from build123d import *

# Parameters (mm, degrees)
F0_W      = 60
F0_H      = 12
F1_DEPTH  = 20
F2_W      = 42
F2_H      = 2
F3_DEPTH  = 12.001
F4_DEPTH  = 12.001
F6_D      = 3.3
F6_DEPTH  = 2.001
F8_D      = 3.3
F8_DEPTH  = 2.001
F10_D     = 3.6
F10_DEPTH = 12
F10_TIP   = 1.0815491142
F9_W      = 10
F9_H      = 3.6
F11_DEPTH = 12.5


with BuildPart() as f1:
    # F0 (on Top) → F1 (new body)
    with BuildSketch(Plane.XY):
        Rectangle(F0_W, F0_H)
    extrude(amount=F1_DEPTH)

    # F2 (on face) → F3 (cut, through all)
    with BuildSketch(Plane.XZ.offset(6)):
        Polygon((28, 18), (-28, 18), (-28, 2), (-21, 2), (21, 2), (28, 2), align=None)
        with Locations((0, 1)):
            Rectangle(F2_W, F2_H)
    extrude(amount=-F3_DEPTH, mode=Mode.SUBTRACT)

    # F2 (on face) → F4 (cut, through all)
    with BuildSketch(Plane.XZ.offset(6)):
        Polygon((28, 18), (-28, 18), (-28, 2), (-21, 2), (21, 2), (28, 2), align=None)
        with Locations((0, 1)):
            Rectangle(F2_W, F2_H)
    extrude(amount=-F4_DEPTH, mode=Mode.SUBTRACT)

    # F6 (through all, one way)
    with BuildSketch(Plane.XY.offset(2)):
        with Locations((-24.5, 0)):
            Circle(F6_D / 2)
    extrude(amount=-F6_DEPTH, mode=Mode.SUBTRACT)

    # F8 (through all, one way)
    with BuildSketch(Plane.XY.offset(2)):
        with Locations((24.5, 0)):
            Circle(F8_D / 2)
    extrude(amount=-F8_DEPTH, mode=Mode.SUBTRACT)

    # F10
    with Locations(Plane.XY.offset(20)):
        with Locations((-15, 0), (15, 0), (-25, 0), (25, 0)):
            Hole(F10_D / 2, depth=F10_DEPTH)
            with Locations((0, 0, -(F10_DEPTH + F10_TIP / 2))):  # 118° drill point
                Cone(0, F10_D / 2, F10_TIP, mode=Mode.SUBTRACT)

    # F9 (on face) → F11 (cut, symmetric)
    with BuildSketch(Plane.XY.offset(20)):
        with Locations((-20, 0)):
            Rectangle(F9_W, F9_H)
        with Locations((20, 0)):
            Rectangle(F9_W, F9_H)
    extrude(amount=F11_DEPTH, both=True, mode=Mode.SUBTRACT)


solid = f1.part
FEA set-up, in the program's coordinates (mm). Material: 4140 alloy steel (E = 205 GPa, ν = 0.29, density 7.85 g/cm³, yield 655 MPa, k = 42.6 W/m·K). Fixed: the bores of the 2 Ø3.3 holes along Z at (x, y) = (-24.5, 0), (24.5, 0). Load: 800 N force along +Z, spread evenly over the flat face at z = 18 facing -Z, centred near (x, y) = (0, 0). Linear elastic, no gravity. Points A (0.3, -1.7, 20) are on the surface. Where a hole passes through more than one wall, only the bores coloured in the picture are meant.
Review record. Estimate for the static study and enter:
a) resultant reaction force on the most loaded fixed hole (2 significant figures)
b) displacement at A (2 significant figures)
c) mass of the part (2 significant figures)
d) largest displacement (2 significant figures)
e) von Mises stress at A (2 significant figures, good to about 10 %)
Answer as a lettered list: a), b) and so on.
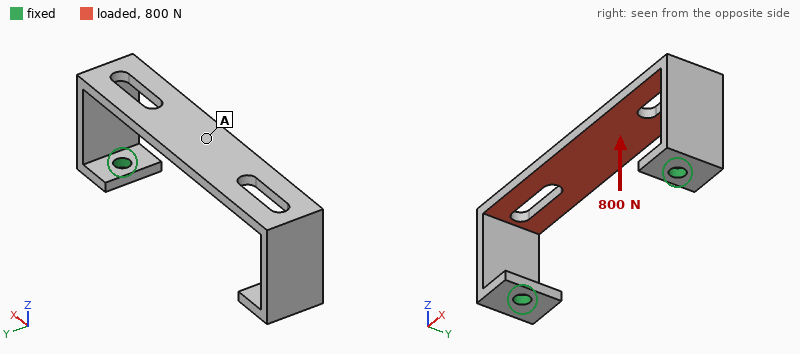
a) 470 N
b) 0.46 mm
c) 19 g
d) 0.47 mm
e) 360 MPa
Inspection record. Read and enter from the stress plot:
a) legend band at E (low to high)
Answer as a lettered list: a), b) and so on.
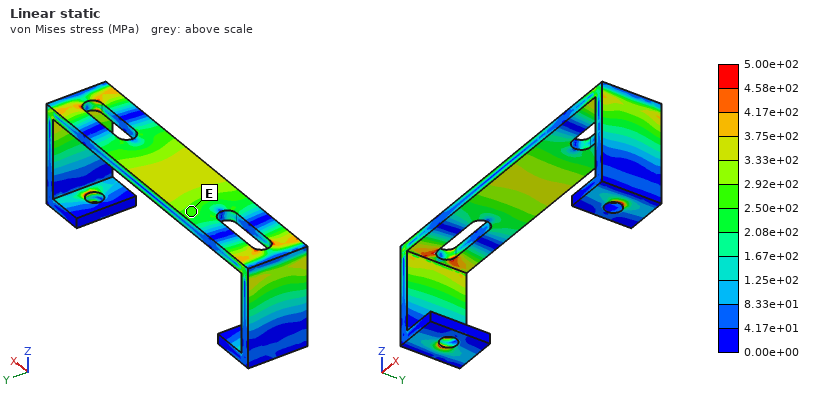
a) 2.50e+02 to 2.92e+02 MPa
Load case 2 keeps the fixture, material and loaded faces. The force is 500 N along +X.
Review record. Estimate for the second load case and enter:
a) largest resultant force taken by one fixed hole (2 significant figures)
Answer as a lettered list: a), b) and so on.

a) 250 N
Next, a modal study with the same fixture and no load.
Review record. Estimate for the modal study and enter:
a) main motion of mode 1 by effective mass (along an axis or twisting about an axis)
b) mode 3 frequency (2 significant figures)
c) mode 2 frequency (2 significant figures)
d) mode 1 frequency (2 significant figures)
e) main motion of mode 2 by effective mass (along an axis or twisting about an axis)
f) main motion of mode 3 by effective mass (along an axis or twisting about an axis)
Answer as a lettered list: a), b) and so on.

a) along X
b) 3000 Hz
c) 2400 Hz
d) 2100 Hz
e) along Z
f) along Y
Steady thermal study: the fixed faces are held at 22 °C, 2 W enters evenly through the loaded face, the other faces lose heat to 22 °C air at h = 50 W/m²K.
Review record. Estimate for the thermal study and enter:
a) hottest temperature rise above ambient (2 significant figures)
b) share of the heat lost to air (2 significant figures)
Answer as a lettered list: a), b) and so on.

a) 21 K
b) 57 %
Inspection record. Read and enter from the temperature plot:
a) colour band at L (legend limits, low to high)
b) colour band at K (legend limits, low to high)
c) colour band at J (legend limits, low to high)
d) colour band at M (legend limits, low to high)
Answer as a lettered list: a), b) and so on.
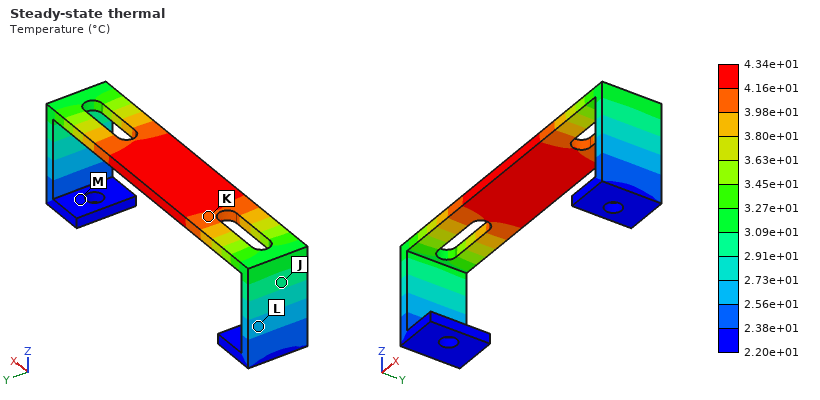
a) 2.56e+01 to 2.73e+01 °C
b) 3.98e+01 to 4.16e+01 °C
c) 2.91e+01 to 3.09e+01 °C
d) 2.20e+01 to 2.38e+01 °C
